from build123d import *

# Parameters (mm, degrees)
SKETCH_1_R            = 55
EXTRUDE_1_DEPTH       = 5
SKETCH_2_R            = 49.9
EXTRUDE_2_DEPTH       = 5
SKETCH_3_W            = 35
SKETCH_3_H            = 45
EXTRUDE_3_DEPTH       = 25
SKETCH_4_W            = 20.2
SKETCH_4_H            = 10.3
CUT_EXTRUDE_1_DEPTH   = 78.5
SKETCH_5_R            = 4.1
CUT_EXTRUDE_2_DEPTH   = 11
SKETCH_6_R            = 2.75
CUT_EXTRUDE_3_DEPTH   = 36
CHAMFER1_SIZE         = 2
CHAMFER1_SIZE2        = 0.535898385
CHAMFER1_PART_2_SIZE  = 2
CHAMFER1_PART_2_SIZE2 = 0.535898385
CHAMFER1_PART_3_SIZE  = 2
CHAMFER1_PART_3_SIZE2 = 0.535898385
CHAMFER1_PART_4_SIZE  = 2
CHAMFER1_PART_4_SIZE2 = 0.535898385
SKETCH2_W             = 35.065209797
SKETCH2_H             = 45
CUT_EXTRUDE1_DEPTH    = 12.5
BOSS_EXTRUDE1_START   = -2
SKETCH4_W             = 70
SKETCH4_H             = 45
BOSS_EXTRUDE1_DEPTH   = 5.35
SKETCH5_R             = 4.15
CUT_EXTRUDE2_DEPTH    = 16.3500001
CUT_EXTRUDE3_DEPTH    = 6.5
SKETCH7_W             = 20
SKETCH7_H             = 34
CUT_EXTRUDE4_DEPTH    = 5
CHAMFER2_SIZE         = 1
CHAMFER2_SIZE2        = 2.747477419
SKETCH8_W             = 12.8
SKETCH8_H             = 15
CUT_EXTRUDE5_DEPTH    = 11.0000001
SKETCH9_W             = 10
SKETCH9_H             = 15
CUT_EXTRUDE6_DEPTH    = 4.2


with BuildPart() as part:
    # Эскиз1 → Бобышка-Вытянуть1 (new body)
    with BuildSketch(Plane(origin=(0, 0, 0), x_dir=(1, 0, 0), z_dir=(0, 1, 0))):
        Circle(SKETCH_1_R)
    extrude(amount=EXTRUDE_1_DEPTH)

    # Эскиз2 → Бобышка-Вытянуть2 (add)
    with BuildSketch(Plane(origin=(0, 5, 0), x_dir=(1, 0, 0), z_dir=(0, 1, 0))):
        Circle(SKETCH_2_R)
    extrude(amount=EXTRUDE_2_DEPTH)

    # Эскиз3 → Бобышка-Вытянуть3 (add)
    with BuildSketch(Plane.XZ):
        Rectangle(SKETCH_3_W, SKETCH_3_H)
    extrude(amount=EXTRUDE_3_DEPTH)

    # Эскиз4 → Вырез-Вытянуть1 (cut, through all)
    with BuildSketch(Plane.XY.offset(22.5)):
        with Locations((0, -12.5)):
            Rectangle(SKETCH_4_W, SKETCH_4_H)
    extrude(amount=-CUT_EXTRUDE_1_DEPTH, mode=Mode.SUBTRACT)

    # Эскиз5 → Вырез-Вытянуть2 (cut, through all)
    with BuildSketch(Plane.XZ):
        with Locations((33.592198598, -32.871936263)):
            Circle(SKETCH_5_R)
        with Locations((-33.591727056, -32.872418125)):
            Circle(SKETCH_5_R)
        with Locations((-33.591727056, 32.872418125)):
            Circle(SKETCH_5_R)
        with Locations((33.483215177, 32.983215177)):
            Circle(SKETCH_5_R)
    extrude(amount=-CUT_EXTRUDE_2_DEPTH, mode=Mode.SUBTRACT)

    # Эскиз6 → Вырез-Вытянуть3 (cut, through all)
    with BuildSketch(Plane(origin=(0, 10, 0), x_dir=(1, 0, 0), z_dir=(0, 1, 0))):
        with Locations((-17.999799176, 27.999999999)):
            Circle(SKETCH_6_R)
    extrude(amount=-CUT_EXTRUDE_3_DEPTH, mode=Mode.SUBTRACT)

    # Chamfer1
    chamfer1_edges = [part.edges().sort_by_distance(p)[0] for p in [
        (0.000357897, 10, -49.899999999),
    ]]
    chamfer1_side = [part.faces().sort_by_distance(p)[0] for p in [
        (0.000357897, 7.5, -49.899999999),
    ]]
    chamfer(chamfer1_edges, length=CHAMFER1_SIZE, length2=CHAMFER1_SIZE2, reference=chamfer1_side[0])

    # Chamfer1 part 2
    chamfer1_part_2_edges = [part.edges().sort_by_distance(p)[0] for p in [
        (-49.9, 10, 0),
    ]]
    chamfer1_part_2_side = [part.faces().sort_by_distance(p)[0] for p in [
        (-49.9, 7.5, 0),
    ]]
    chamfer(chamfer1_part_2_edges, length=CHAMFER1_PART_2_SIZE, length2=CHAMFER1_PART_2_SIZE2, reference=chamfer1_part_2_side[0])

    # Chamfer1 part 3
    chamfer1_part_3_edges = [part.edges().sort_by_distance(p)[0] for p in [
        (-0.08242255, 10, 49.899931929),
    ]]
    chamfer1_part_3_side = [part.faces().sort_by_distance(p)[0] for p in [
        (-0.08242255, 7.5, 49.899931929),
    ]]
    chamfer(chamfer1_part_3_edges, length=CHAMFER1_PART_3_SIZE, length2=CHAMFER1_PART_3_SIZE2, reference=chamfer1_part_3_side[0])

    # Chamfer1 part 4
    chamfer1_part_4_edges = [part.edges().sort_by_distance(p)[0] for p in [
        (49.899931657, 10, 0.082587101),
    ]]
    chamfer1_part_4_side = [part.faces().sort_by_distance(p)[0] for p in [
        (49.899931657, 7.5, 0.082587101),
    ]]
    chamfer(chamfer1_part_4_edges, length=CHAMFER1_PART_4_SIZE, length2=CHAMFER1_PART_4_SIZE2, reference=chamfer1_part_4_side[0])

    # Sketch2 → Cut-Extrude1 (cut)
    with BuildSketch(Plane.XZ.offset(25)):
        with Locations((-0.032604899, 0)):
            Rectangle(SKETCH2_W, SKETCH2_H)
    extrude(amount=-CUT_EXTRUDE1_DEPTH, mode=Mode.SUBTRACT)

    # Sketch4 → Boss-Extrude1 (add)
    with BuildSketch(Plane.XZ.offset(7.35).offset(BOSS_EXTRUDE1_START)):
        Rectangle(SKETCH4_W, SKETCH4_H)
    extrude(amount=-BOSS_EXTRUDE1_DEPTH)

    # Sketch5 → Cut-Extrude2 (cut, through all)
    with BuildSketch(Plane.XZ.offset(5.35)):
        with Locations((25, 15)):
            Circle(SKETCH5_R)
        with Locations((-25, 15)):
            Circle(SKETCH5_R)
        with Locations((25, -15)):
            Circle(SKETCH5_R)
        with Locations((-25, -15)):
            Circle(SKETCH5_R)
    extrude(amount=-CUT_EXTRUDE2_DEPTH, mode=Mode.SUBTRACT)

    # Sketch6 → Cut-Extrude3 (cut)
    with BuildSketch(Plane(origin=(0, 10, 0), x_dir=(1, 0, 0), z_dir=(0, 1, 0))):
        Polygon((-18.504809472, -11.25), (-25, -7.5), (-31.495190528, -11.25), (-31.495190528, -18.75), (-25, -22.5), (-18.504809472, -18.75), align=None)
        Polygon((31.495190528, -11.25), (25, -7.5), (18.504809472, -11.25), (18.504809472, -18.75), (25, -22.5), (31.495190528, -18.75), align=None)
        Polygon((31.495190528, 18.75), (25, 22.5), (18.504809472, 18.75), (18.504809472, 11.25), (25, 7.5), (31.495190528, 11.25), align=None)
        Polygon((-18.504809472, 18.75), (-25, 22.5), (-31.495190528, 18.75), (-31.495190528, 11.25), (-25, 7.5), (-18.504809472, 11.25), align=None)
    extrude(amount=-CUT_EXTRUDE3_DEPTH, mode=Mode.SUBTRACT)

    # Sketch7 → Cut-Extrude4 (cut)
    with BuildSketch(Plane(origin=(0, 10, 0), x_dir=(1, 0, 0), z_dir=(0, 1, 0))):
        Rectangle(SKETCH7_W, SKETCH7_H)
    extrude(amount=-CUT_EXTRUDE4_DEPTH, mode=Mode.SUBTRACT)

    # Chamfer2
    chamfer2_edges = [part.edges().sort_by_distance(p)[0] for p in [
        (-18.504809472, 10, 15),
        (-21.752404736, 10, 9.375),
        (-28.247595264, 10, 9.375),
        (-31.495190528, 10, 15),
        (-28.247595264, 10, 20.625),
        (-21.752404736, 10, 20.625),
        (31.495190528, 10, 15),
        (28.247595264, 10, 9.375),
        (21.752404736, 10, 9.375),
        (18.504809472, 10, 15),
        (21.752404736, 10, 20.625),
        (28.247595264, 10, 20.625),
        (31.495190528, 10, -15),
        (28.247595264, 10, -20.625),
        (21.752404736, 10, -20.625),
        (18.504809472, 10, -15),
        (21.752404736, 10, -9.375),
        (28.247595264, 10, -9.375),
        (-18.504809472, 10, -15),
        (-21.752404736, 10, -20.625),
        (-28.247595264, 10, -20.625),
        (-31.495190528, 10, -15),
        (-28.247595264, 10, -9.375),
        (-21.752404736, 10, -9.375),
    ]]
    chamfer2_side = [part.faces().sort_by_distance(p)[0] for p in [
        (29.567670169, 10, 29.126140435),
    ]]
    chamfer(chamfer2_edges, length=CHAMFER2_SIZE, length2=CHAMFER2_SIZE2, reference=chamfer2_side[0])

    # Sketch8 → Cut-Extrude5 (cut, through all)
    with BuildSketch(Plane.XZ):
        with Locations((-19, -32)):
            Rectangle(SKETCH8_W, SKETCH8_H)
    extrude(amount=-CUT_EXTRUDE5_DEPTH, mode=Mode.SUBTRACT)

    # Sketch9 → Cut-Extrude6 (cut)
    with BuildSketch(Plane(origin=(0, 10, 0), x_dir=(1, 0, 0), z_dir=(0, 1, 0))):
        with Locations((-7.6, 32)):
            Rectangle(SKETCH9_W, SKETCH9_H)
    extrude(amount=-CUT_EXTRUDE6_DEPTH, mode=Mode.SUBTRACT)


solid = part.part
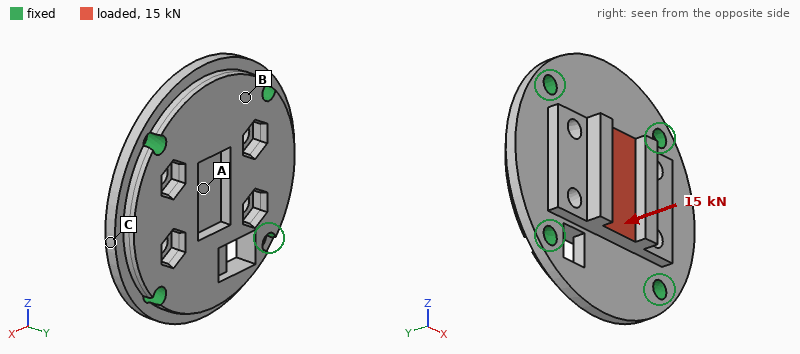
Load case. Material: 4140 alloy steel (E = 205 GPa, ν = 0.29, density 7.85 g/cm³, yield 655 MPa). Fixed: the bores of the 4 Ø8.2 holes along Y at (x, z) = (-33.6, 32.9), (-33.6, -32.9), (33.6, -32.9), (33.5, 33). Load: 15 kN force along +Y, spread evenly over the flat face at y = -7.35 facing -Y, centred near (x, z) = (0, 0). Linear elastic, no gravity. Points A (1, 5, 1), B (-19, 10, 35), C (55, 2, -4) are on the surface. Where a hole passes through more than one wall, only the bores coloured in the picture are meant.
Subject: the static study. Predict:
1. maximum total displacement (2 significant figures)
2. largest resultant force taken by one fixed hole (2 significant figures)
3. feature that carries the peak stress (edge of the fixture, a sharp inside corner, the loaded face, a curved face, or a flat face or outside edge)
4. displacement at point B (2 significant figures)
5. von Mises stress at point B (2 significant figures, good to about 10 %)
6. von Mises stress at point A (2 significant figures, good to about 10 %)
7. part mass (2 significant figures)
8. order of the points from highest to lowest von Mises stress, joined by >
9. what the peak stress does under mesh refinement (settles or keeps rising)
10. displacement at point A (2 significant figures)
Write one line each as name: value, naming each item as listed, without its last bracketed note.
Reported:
maximum total displacement: 24 µm
largest resultant force taken by one fixed hole: 5.0 kN
feature that carries the peak stress: edge of the fixture
displacement at point B: 6.0 µm
von Mises stress at point B: 22 MPa
von Mises stress at point A: 45 MPa
part mass: 750 g
order of the points from highest to lowest von Mises stress, joined by >: A > B > C
what the peak stress does under mesh refinement: keeps rising
displacement at point A: 23 µm
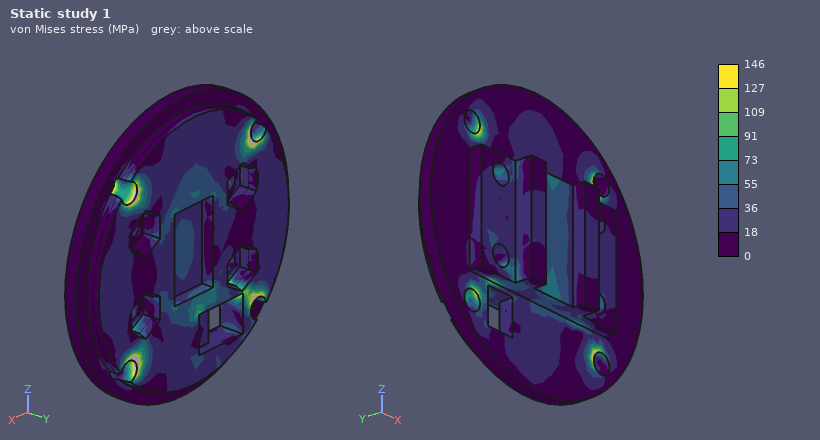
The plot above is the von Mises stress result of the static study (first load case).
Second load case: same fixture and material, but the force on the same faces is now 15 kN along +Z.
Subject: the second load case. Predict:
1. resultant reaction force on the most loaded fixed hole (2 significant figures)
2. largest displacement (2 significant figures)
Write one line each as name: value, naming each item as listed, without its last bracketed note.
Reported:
resultant reaction force on the most loaded fixed hole: 4.8 kN
largest displacement: 11 µm
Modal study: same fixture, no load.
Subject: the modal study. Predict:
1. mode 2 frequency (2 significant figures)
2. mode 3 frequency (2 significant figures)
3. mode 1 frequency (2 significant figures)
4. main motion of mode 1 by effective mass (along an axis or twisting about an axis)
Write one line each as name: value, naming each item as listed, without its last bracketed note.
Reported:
mode 2 frequency: 9100 Hz
mode 3 frequency: 10 kHz
mode 1 frequency: 7700 Hz
main motion of mode 1 by effective mass: along Y
